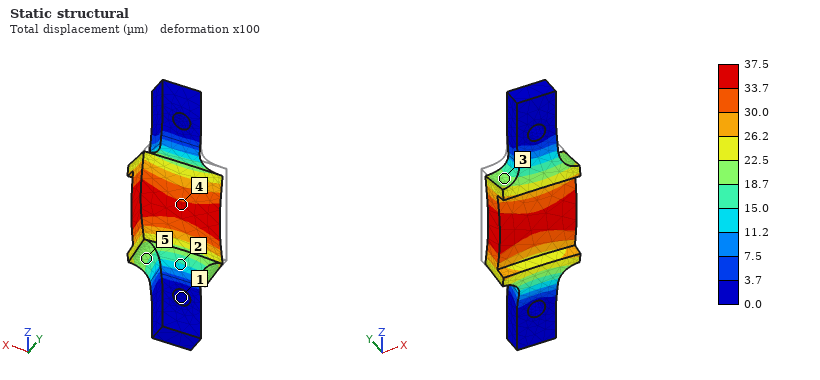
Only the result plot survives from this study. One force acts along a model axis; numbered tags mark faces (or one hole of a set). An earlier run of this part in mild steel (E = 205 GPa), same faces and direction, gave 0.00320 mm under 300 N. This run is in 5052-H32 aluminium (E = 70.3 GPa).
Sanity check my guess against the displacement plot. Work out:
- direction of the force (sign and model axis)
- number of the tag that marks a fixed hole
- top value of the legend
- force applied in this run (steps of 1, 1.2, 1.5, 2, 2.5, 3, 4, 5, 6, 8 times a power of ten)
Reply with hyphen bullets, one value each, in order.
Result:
- -Y
- 1
- 37.5 µm
- 1.2 kN
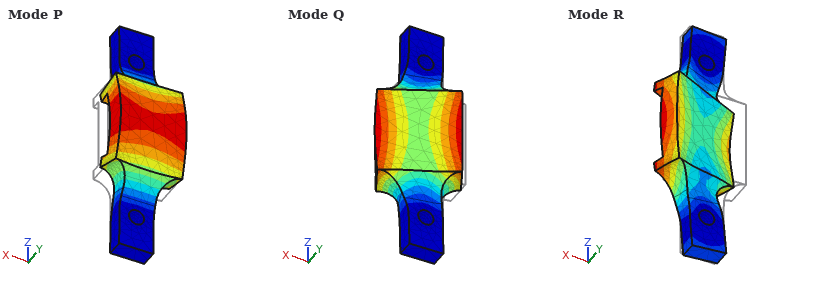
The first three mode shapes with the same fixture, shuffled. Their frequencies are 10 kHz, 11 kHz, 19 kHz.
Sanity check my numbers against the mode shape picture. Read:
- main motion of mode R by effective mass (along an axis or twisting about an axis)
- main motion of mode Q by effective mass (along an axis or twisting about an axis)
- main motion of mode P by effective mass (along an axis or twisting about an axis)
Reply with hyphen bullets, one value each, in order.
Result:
- along X
- along X
- along Y
